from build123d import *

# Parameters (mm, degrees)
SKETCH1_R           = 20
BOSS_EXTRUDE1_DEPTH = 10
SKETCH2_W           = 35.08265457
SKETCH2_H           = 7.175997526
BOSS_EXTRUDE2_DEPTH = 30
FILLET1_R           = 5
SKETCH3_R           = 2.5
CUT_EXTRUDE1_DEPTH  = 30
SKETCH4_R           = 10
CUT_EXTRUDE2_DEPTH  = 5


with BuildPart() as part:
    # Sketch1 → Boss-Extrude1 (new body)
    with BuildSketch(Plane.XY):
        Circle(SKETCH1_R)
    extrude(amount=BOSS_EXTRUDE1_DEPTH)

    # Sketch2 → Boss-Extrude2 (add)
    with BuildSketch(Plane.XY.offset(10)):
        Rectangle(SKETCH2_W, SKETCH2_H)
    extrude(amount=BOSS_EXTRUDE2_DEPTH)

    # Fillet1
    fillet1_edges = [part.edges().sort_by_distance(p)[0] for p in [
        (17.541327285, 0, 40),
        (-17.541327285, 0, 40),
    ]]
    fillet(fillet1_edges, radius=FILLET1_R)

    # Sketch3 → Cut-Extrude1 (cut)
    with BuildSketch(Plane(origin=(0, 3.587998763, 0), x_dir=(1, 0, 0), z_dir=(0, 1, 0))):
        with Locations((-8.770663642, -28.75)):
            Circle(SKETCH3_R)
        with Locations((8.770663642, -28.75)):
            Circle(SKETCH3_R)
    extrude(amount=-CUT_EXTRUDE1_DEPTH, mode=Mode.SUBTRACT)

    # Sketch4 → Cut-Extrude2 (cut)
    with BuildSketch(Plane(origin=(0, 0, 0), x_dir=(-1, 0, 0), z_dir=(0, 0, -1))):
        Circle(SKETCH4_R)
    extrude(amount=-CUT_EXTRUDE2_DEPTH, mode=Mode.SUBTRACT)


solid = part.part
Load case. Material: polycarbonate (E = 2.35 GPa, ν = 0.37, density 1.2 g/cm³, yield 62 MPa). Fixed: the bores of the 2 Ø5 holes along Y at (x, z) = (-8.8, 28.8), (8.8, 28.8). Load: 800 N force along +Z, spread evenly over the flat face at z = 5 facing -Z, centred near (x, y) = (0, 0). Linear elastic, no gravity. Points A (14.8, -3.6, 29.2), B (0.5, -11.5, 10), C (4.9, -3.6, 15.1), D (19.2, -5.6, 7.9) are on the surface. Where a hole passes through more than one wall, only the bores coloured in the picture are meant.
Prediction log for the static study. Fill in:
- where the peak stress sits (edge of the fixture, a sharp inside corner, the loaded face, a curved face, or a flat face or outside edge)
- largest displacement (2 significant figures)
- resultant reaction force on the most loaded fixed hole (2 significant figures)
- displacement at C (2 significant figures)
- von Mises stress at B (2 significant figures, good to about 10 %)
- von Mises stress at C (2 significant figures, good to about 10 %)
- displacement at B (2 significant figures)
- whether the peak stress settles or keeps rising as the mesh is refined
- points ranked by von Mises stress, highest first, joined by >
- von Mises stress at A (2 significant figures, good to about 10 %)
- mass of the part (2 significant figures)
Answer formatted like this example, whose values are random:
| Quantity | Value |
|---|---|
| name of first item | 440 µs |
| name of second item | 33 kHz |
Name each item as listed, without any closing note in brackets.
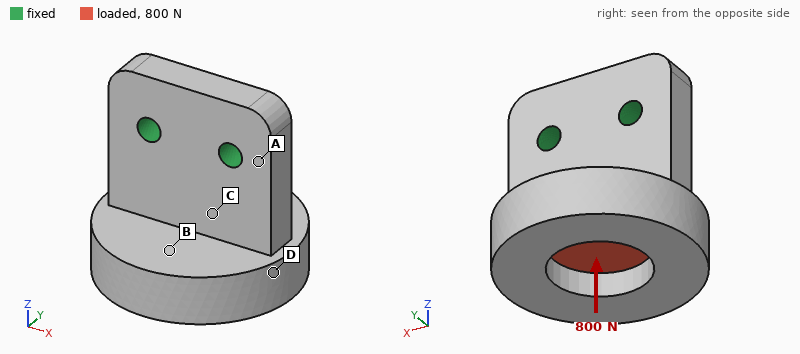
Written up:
| Quantity | Value |
|---|---|
| where the peak stress sits | edge of the fixture |
| largest displacement | 53 µm |
| resultant reaction force on the most loaded fixed hole | 410 N |
| displacement at C | 24 µm |
| von Mises stress at B | 2.3 MPa |
| von Mises stress at C | 4.4 MPa |
| displacement at B | 48 µm |
| whether the peak stress settles or keeps rising as the mesh is refined | keeps rising |
| points ranked by von Mises stress, highest first, joined by > | C > B > A > D |
| von Mises stress at A | 1.4 MPa |
| mass of the part | 22 g |
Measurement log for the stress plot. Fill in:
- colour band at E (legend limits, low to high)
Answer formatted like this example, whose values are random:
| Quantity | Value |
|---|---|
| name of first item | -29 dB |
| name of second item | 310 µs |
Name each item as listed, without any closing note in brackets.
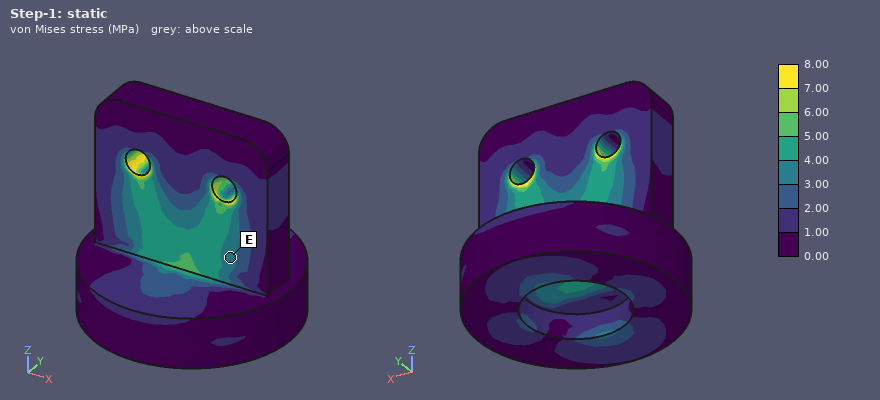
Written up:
| Quantity | Value |
|---|---|
| colour band at E | 3.00 to 4.00 MPa |
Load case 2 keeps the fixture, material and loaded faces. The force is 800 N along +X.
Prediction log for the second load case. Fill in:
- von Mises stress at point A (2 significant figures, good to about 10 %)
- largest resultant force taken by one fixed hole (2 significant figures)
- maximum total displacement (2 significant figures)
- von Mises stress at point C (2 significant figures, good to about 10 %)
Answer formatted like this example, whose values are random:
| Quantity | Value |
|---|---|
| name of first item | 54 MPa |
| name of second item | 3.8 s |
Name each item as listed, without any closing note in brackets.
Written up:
| Quantity | Value |
|---|---|
| von Mises stress at point A | 5.8 MPa |
| largest resultant force taken by one fixed hole | 970 N |
| maximum total displacement | 0.23 mm |
| von Mises stress at point C | 8.4 MPa |
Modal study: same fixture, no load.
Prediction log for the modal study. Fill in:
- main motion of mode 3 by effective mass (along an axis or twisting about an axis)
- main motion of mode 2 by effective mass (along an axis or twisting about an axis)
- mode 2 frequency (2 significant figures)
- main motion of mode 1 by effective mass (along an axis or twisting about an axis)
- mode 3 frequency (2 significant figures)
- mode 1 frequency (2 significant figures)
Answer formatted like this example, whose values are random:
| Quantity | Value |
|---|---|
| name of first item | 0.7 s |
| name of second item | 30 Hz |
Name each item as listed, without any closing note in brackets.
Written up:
| Quantity | Value |
|---|---|
| main motion of mode 3 by effective mass | along X |
| main motion of mode 2 by effective mass | twisting about Z |
| mode 2 frequency | 1700 Hz |
| main motion of mode 1 by effective mass | along Y |
| mode 3 frequency | 2600 Hz |
| mode 1 frequency | 880 Hz |
